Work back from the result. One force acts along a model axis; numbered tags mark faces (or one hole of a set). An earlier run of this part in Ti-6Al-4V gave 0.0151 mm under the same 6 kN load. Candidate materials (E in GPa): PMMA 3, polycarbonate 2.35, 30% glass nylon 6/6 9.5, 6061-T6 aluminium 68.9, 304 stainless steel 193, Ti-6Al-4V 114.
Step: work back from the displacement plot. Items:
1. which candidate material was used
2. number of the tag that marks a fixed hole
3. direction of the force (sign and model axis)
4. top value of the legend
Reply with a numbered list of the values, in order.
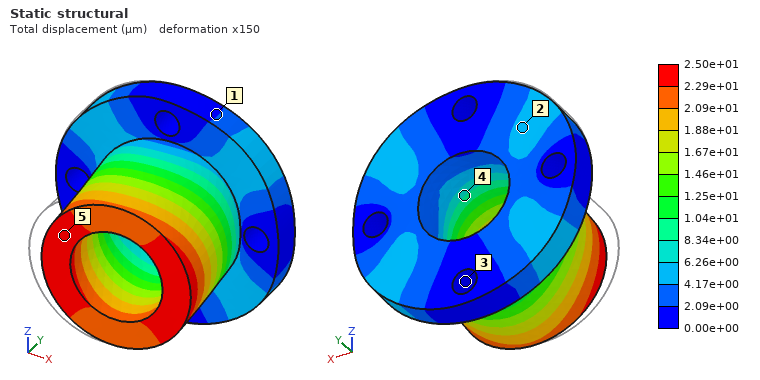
1. 6061-T6 aluminium
2. 3
3. +X
4. 2.50e+01 µm
